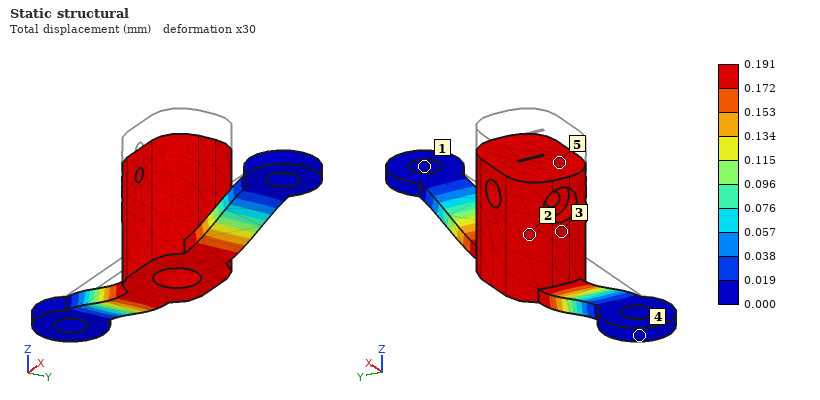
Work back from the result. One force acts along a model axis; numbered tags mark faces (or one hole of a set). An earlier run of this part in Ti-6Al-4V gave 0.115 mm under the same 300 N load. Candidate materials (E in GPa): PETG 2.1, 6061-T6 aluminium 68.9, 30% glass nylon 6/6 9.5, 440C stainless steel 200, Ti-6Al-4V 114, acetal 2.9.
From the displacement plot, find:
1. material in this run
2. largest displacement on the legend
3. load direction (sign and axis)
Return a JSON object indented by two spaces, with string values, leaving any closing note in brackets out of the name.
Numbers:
{
  "material in this run": "6061-T6 aluminium",
  "largest displacement on the legend": "0.191 mm",
  "load direction": "-Z"
}
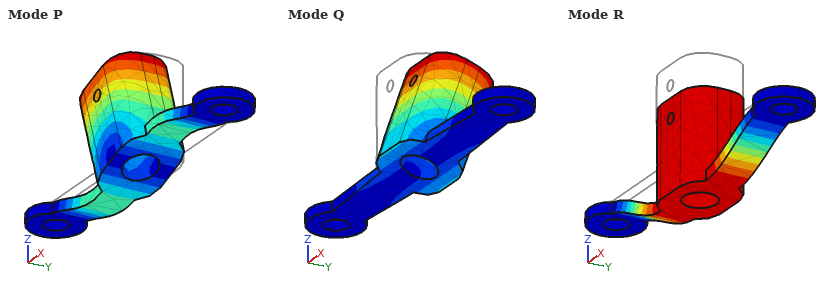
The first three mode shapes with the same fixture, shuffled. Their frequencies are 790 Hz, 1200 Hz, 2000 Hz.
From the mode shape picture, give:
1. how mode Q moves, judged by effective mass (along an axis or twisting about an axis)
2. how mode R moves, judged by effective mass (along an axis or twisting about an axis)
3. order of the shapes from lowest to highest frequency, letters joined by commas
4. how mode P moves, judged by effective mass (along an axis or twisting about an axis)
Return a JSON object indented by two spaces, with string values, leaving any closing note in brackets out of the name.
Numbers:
{
  "how mode Q moves, judged by effective mass": "along Y",
  "how mode R moves, judged by effective mass": "along Z",
  "order of the shapes from lowest to highest frequency, letters joined by commas": "Q, R, P",
  "how mode P moves, judged by effective mass": "along X"
}
